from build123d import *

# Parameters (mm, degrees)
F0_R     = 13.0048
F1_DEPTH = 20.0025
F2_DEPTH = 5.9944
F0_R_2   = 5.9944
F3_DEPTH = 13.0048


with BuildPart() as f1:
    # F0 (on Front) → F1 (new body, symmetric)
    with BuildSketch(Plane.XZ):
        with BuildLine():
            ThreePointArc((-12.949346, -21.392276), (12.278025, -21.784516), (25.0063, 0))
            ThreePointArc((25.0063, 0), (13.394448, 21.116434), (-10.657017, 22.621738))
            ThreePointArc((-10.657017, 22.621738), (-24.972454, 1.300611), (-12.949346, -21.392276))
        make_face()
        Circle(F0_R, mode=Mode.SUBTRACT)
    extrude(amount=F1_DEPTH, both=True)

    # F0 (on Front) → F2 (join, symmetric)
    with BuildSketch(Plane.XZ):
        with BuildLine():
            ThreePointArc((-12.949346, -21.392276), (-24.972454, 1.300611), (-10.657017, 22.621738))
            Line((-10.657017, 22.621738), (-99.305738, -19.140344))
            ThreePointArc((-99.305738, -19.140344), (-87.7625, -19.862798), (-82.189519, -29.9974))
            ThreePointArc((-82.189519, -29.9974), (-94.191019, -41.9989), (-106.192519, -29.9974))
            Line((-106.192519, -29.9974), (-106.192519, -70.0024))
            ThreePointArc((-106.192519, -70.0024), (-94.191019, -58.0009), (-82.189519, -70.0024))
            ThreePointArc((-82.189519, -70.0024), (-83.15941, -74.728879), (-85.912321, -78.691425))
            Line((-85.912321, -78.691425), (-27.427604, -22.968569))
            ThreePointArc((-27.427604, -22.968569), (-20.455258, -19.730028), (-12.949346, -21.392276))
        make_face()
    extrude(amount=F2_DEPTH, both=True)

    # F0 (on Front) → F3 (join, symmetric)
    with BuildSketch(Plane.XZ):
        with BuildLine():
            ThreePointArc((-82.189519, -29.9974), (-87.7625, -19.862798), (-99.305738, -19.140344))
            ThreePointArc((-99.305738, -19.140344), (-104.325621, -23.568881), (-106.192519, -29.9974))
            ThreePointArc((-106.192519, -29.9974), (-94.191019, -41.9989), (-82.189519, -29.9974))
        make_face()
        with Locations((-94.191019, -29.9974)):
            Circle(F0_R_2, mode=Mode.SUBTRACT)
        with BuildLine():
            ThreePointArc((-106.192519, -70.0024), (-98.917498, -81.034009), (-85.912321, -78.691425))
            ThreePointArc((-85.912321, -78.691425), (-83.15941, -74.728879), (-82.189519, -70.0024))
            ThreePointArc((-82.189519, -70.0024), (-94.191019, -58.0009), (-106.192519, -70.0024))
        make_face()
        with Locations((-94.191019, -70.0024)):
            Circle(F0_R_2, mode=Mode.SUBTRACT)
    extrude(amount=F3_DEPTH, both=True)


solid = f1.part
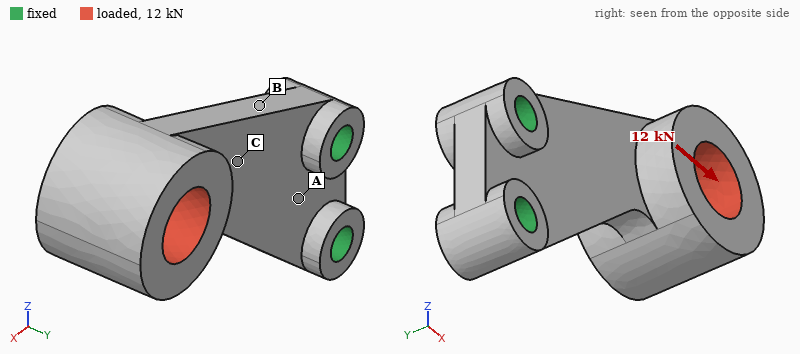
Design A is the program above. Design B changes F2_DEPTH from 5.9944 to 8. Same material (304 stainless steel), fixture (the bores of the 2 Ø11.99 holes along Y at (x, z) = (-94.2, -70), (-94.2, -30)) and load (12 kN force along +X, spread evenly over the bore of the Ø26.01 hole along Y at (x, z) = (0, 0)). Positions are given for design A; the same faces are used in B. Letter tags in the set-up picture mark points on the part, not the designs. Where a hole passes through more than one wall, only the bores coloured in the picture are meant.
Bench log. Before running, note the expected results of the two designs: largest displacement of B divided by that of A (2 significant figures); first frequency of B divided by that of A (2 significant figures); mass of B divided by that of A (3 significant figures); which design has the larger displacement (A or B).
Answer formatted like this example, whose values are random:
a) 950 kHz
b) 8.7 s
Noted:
a) 0.76
b) 1.5
c) 1.12
d) A
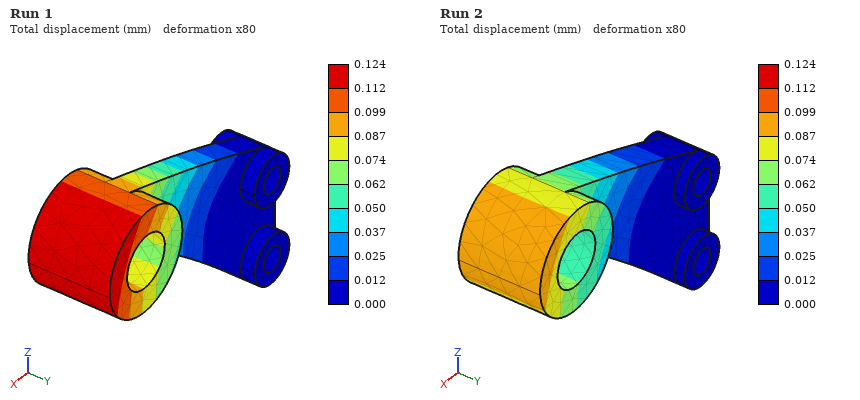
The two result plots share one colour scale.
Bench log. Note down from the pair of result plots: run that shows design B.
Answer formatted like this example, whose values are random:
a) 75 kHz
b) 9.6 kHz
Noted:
a) Run 2
